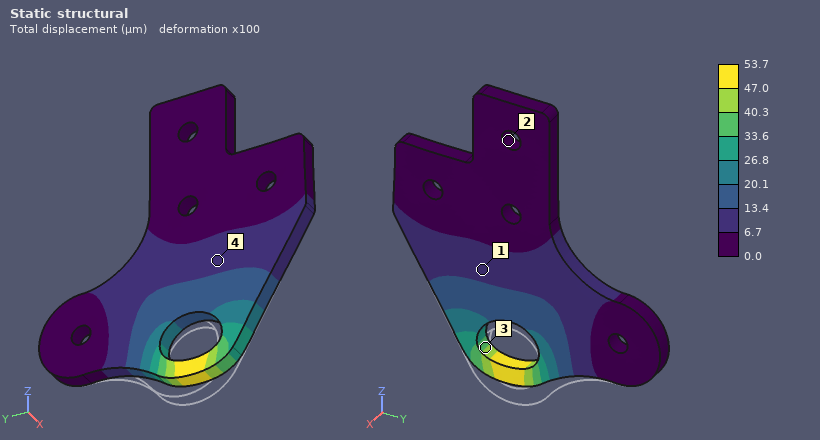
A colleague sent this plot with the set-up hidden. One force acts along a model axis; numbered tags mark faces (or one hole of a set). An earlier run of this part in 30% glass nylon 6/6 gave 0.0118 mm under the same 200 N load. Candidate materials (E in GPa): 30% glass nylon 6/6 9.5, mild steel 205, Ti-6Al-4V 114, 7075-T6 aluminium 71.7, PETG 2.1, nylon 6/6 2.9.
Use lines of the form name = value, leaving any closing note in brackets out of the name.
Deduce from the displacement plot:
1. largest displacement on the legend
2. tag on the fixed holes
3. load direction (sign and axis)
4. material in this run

largest displacement on the legend = 53.7 µm
tag on the fixed holes = 2
load direction = +Z
material in this run = PETG
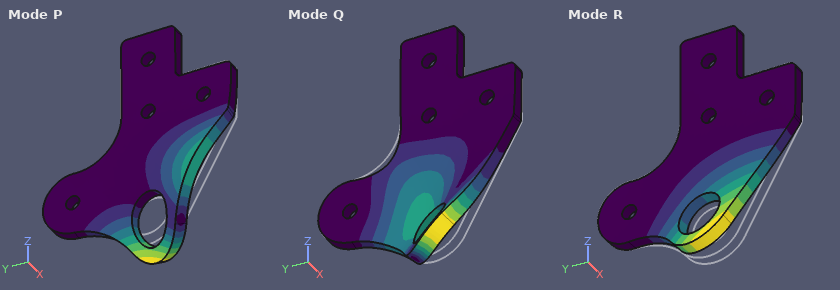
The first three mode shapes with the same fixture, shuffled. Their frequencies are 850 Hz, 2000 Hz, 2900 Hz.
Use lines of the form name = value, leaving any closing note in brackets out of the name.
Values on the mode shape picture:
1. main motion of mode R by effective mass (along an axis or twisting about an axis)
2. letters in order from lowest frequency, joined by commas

main motion of mode R by effective mass = along X
letters in order from lowest frequency, joined by commas = R, P, Q
